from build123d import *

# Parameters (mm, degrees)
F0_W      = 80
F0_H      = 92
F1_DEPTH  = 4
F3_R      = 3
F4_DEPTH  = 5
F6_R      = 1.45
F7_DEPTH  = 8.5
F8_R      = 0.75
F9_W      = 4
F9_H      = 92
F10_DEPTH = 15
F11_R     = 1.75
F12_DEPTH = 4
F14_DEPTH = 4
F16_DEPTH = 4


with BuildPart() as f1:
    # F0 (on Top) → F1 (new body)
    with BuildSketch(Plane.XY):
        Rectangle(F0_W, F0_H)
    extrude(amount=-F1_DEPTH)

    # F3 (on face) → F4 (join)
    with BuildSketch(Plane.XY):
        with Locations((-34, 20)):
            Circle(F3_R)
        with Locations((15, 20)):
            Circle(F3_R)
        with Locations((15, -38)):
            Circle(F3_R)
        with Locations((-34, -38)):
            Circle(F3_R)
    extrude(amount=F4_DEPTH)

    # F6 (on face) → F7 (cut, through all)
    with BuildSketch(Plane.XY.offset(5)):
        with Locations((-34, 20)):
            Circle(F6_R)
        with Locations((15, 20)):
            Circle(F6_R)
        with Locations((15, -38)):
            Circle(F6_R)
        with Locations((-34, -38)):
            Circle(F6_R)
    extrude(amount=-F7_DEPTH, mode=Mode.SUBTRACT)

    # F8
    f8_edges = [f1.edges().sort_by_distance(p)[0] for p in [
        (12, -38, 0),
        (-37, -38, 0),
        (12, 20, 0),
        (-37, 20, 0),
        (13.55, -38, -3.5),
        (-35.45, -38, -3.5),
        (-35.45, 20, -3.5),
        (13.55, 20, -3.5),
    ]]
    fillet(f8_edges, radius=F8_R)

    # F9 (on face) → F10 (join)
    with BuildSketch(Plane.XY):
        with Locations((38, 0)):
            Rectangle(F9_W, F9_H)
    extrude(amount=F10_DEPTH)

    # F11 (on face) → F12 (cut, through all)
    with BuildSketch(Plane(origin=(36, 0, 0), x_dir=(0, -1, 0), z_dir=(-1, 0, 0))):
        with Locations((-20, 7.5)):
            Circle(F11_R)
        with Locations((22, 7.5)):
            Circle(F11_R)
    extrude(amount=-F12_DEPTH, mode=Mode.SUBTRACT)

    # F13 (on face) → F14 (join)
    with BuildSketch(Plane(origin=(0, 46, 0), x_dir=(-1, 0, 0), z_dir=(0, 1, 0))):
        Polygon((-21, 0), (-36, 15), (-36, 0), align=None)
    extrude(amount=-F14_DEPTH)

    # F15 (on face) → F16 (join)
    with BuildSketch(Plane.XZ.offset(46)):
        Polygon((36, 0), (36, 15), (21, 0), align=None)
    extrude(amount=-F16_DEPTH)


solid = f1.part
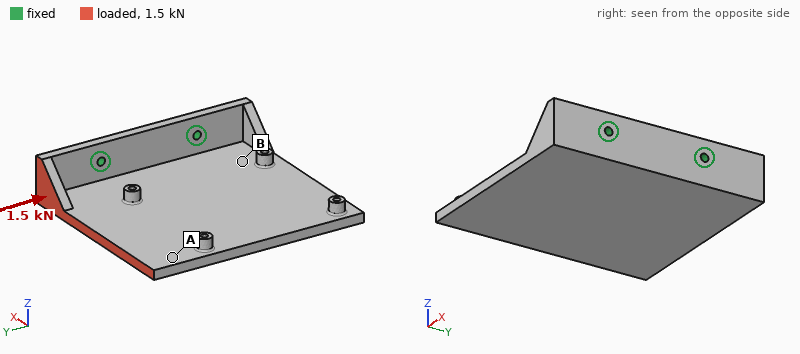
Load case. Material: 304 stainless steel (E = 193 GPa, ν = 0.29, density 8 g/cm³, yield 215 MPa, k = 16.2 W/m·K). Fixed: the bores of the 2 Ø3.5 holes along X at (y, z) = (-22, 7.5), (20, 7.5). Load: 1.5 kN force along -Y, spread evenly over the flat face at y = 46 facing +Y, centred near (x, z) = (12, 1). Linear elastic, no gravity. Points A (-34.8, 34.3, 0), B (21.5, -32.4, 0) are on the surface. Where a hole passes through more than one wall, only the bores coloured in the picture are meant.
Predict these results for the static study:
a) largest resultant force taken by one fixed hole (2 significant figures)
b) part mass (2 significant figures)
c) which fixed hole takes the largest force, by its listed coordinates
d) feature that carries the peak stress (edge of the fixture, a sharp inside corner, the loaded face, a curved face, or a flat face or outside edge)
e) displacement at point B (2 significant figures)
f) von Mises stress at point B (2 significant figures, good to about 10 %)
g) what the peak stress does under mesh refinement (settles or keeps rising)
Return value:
1.3 kN
290 g
(20, 7.5)
edge of the fixture
20 µm
16 MPa
keeps rising
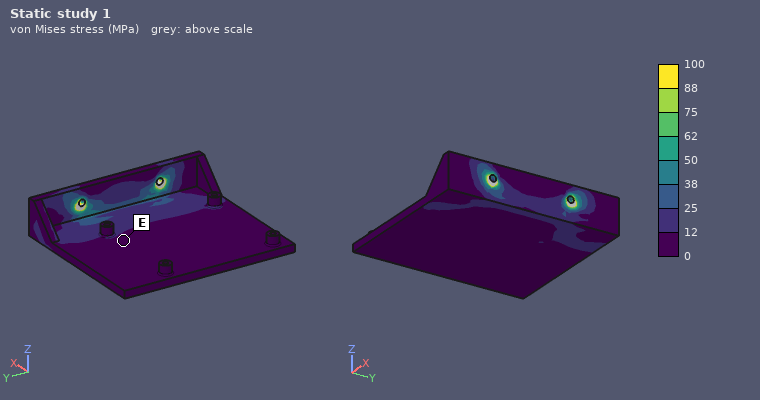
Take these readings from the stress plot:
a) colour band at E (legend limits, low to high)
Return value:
0 to 12 MPa
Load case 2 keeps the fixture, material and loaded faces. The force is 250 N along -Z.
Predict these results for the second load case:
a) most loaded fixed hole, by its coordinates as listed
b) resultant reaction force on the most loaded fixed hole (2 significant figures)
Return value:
(20, 7.5)
400 N
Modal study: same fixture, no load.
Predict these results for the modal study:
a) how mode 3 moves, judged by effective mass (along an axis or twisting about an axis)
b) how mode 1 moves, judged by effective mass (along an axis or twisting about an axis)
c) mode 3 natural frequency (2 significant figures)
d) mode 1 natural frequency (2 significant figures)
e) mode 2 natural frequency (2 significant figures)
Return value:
along Y
along Z
1900 Hz
420 Hz
1000 Hz
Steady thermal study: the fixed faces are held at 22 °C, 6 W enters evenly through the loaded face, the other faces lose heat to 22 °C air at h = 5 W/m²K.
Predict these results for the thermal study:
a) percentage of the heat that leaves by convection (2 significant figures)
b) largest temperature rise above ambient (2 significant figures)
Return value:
33 %
48 K
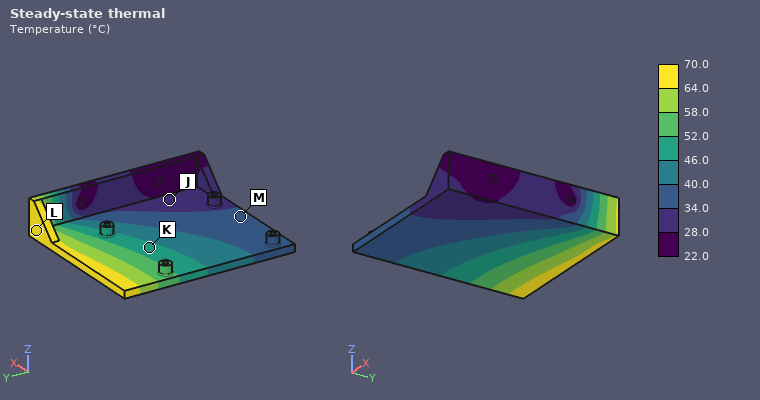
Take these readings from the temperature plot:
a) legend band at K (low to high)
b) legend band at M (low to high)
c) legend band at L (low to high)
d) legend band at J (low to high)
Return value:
46.0 to 52.0 °C
34.0 to 40.0 °C
64.0 to 70.0 °C
28.0 to 34.0 °C
